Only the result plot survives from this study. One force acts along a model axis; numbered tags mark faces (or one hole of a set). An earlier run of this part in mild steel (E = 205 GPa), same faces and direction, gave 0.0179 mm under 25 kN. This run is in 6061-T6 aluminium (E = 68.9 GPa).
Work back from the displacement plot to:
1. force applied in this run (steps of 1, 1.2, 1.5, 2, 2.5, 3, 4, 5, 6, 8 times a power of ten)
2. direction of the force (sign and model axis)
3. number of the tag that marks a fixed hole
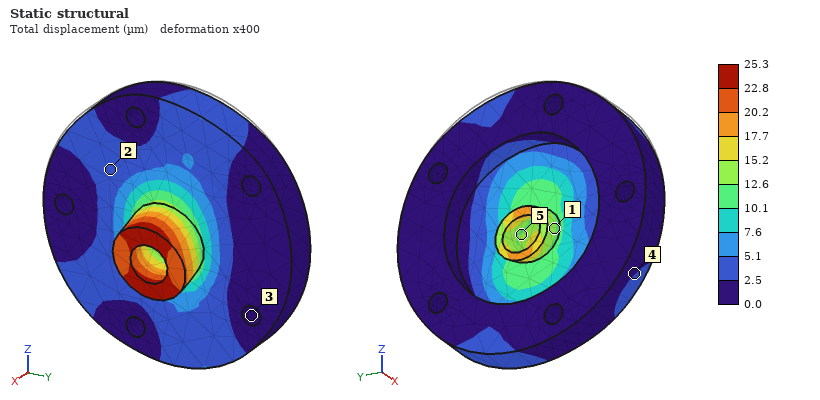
12 kN
-Z
3
